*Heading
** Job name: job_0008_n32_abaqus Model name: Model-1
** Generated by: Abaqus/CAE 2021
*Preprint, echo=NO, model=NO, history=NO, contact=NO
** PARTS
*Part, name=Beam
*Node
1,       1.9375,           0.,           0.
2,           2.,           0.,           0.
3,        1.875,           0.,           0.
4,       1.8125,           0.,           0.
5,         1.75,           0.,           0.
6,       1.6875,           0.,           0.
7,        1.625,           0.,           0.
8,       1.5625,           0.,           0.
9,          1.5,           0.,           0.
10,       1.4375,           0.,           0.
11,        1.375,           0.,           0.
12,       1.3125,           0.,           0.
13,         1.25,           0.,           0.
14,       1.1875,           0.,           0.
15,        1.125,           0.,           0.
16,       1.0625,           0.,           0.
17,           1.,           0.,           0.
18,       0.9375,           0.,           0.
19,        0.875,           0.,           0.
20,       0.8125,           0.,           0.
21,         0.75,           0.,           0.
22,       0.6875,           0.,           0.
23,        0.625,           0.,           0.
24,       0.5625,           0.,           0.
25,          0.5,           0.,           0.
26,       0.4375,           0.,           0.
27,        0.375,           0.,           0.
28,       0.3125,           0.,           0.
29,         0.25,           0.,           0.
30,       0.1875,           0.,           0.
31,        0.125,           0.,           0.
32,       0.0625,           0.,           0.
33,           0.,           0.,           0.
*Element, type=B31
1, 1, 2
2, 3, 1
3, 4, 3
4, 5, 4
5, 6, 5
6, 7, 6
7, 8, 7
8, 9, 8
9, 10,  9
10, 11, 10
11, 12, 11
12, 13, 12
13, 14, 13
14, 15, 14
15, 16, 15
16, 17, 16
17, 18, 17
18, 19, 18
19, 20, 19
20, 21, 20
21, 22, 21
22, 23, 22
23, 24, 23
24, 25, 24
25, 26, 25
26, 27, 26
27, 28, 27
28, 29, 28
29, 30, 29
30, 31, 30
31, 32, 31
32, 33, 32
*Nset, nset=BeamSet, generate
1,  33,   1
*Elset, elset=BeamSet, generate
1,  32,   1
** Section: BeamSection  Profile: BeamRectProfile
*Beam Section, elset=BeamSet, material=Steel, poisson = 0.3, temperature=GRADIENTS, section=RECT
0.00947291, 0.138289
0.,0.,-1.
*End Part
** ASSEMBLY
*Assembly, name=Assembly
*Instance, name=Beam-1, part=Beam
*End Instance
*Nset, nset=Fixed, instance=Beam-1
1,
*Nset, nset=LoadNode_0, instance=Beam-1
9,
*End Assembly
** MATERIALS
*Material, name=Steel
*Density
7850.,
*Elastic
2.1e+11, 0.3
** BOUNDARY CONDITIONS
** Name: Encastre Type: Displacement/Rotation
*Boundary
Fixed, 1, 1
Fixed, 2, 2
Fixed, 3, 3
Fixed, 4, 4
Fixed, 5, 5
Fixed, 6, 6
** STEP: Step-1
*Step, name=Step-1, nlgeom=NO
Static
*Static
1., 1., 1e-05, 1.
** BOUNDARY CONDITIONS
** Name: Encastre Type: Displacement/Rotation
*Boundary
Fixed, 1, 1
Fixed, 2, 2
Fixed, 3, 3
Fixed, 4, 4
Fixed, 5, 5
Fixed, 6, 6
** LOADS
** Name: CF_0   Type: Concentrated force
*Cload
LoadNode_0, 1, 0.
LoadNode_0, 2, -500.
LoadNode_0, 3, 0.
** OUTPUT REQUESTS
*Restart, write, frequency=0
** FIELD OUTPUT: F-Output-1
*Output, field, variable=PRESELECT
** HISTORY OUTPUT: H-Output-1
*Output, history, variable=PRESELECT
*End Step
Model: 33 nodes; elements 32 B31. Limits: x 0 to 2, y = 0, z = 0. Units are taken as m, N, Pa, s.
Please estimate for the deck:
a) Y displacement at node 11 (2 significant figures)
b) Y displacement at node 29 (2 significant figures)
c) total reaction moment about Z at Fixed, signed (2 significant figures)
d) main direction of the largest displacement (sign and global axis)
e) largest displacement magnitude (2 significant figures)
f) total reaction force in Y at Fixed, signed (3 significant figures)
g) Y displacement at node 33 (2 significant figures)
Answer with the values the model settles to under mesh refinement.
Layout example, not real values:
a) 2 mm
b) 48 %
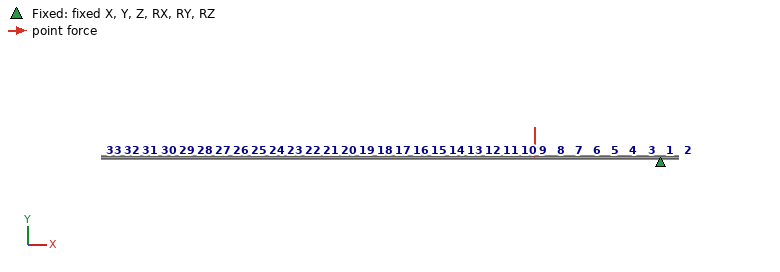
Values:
a) -4.8e-05 m
b) -1.7e-04 m
c) -220 N·m
d) -Y
e) 2.0e-04 m
f) 500 N
g) -2.0e-04 m
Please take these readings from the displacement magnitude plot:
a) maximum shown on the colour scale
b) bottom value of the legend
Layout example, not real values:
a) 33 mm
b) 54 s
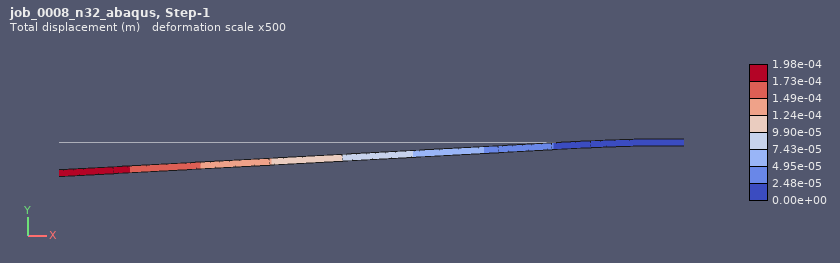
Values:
a) 1.98e-04 m
b) 0.00e+00 m
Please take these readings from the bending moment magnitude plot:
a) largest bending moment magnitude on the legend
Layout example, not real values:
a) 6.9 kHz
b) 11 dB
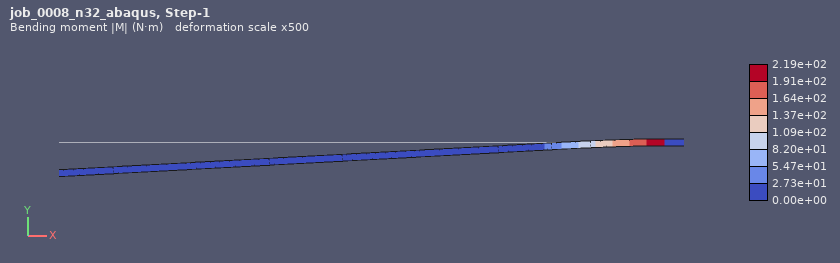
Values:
a) 2.19e+02 N·m
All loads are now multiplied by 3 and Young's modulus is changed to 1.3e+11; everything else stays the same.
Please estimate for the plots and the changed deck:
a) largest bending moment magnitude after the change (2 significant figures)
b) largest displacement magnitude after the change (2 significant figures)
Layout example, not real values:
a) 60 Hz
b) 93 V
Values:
a) 660 N·m
b) 9.6e-04 m
